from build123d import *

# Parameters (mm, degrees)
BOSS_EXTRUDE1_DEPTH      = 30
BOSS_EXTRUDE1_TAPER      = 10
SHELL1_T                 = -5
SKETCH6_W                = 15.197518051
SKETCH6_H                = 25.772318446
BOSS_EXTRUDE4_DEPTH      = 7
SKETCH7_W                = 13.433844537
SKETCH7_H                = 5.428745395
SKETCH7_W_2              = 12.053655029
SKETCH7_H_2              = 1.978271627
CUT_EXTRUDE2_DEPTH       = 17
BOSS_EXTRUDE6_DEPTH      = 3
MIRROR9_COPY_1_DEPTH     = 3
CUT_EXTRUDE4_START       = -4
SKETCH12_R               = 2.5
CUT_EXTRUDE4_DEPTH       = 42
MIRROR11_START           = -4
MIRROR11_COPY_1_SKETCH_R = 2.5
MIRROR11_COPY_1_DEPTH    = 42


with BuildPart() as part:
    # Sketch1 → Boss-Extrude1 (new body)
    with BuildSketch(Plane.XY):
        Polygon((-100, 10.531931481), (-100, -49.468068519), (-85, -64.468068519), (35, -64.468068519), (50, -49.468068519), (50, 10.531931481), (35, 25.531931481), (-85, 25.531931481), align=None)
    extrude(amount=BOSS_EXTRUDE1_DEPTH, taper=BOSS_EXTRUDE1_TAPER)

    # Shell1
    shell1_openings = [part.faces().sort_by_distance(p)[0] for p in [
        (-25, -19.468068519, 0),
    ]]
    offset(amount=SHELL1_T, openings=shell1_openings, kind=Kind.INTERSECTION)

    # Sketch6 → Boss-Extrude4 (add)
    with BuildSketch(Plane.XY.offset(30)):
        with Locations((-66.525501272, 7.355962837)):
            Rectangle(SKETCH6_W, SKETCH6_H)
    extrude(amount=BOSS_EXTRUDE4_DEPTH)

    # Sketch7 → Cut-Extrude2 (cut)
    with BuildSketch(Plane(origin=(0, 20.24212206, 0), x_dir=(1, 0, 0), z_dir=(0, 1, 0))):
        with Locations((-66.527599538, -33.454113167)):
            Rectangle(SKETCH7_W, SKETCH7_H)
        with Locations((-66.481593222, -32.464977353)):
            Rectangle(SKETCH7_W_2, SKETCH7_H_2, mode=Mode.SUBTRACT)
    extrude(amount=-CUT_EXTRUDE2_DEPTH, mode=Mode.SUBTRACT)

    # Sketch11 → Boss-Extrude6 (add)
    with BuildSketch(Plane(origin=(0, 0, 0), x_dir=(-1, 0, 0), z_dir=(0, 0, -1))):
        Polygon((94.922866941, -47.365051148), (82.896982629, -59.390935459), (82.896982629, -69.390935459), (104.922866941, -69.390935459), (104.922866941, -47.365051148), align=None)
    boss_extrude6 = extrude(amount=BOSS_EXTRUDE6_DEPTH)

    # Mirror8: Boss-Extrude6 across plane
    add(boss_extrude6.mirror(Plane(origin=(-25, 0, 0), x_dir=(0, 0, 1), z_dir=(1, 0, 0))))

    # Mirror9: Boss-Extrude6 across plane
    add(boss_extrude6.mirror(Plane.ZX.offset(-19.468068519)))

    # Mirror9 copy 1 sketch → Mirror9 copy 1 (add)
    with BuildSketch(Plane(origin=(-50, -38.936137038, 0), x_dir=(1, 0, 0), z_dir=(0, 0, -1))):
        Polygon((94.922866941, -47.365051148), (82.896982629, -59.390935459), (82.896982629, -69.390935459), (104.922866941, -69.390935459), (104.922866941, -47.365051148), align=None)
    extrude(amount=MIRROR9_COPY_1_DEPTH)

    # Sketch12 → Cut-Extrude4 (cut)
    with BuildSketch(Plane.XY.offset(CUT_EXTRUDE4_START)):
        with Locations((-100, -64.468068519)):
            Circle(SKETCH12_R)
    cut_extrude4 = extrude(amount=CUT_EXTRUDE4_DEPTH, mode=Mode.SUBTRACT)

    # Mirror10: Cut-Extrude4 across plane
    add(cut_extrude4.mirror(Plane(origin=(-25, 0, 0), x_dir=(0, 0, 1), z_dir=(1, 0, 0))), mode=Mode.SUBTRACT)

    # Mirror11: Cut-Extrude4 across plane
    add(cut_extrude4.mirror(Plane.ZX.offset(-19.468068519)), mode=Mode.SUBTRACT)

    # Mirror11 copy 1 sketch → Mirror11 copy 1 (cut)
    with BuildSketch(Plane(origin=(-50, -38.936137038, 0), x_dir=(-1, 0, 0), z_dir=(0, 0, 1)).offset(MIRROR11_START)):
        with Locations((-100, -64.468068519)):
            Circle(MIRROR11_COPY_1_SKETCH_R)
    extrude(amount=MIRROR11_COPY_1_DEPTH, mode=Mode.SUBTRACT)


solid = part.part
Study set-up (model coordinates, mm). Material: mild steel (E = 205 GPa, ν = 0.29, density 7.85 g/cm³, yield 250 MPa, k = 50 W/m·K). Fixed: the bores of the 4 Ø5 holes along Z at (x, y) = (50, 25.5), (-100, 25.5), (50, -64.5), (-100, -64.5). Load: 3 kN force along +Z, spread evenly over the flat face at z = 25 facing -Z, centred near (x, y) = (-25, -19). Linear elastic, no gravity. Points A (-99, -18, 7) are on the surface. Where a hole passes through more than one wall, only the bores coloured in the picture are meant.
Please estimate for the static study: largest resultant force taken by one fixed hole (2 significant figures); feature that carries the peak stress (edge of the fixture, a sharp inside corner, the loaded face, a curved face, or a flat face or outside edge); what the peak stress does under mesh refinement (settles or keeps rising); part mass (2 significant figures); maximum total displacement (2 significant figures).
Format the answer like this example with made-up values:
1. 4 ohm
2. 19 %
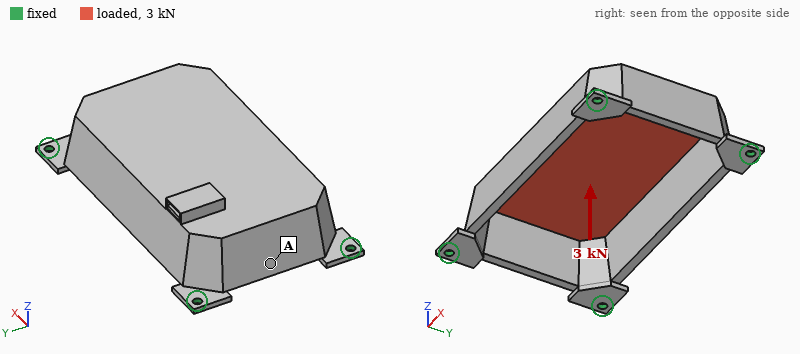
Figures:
1. 1.1 kN
2. edge of the fixture
3. keeps rising
4. 890 g
5. 43 µm
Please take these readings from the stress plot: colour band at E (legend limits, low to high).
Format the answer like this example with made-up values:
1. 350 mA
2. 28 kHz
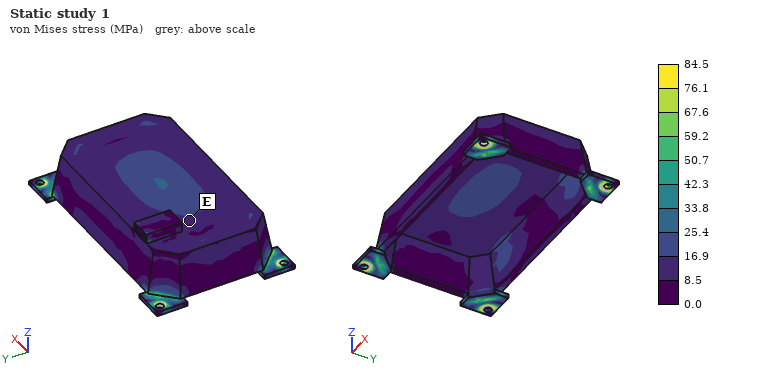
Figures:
1. 8.5 to 16.9 MPa
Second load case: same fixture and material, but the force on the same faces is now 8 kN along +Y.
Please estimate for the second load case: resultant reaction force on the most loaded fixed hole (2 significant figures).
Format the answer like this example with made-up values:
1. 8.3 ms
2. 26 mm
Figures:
1. 2.4 kN
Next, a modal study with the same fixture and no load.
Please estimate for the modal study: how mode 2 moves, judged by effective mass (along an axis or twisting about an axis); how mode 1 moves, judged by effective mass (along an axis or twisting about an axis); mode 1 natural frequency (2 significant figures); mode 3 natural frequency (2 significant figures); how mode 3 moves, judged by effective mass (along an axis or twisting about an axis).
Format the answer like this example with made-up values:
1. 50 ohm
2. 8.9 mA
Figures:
1. along Y
2. along Z
3. 2200 Hz
4. 3100 Hz
5. along Y
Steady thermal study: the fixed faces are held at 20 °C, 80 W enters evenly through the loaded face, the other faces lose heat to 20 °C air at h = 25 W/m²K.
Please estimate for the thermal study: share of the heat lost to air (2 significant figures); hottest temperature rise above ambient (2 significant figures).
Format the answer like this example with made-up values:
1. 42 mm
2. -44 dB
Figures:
1. 65 %
2. 76 K
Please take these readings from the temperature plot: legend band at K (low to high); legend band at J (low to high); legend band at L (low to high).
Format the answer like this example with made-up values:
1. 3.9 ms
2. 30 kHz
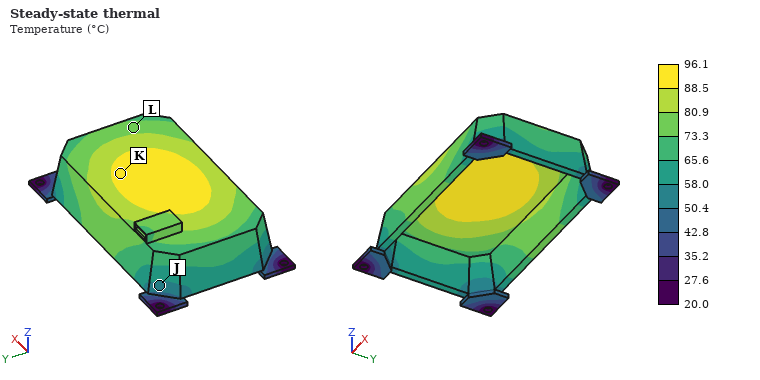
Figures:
1. 88.5 to 96.1 °C
2. 50.4 to 58.0 °C
3. 73.3 to 80.9 °C
